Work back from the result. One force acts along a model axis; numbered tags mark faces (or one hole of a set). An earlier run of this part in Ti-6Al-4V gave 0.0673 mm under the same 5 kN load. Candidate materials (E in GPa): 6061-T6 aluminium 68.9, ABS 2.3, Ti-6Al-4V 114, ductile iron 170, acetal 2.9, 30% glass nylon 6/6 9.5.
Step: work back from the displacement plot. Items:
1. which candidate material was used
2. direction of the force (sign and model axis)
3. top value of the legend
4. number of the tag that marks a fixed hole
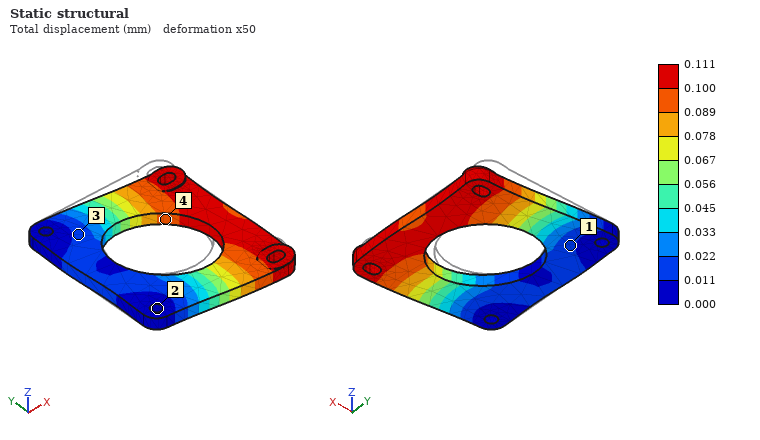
6061-T6 aluminium
-Y
0.111 mm
2
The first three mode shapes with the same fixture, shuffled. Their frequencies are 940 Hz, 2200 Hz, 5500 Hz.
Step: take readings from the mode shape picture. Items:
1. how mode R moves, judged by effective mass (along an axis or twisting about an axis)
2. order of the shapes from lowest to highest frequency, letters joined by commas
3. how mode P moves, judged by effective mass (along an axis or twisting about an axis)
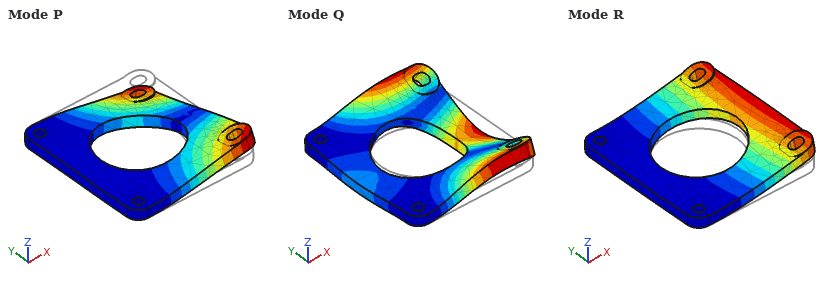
along Z
R, P, Q
twisting about X
